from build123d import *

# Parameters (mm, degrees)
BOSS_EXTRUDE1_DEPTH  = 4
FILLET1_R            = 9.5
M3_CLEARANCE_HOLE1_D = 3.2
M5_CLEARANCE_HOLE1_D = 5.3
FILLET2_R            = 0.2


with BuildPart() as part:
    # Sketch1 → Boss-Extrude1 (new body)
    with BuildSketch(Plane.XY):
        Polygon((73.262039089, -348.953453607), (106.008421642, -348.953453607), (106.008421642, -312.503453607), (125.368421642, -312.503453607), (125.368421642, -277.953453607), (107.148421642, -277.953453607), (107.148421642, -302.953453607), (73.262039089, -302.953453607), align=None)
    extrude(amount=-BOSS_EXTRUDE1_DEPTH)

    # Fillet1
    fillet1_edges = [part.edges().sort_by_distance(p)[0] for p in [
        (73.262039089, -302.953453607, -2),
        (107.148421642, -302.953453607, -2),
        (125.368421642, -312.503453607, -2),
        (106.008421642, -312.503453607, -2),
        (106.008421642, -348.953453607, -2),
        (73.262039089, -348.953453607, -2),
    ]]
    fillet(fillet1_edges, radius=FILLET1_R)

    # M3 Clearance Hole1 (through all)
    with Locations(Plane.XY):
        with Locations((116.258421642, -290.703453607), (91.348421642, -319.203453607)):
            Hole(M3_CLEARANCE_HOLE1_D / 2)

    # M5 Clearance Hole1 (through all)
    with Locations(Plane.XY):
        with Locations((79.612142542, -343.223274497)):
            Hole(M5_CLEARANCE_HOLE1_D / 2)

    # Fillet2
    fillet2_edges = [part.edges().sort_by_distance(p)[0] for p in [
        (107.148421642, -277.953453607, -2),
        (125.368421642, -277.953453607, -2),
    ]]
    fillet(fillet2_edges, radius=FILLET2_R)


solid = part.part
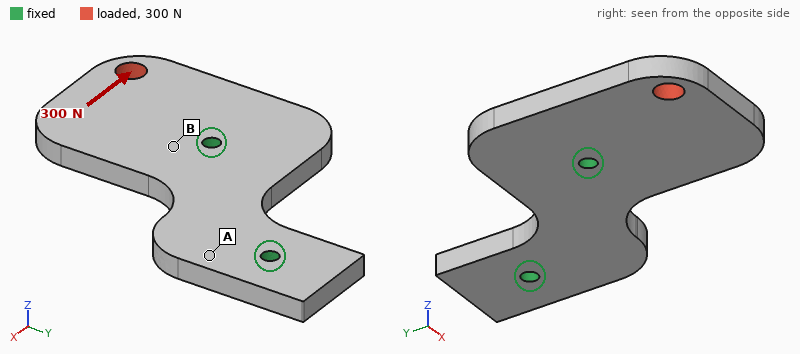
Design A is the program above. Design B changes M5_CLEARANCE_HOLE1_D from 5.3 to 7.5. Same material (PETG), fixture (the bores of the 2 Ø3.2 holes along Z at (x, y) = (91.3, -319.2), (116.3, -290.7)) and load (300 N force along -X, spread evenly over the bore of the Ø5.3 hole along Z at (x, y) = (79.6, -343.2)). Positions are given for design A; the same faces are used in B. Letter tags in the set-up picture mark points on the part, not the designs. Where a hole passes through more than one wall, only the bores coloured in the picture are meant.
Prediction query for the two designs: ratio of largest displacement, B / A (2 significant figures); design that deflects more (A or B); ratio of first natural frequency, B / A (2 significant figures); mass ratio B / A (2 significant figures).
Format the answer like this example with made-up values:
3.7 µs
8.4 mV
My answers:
1.1
B
1.0
0.99
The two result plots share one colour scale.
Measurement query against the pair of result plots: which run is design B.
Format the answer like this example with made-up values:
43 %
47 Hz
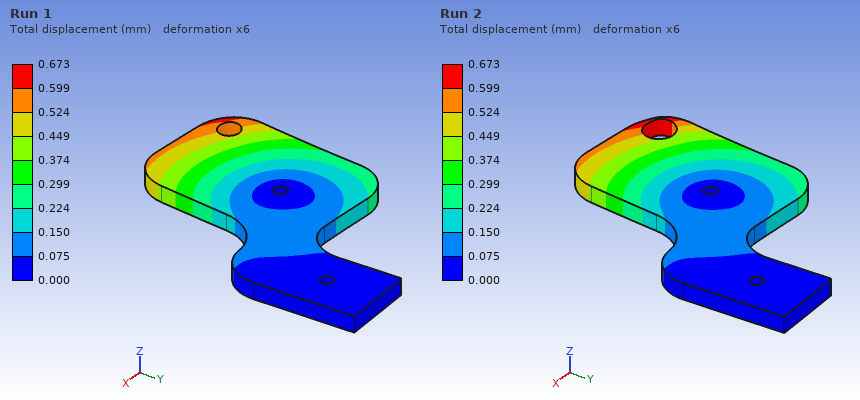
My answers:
Run 2
